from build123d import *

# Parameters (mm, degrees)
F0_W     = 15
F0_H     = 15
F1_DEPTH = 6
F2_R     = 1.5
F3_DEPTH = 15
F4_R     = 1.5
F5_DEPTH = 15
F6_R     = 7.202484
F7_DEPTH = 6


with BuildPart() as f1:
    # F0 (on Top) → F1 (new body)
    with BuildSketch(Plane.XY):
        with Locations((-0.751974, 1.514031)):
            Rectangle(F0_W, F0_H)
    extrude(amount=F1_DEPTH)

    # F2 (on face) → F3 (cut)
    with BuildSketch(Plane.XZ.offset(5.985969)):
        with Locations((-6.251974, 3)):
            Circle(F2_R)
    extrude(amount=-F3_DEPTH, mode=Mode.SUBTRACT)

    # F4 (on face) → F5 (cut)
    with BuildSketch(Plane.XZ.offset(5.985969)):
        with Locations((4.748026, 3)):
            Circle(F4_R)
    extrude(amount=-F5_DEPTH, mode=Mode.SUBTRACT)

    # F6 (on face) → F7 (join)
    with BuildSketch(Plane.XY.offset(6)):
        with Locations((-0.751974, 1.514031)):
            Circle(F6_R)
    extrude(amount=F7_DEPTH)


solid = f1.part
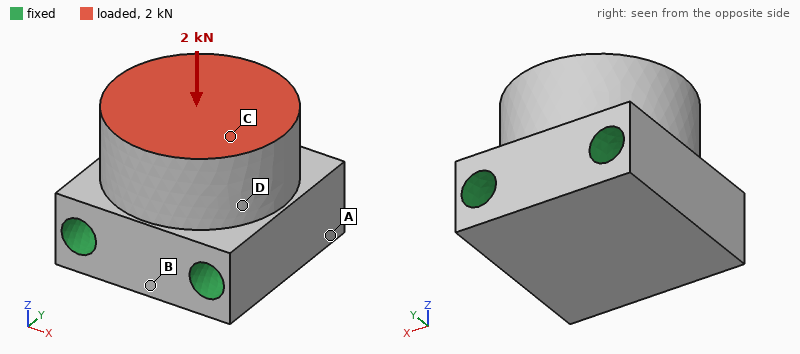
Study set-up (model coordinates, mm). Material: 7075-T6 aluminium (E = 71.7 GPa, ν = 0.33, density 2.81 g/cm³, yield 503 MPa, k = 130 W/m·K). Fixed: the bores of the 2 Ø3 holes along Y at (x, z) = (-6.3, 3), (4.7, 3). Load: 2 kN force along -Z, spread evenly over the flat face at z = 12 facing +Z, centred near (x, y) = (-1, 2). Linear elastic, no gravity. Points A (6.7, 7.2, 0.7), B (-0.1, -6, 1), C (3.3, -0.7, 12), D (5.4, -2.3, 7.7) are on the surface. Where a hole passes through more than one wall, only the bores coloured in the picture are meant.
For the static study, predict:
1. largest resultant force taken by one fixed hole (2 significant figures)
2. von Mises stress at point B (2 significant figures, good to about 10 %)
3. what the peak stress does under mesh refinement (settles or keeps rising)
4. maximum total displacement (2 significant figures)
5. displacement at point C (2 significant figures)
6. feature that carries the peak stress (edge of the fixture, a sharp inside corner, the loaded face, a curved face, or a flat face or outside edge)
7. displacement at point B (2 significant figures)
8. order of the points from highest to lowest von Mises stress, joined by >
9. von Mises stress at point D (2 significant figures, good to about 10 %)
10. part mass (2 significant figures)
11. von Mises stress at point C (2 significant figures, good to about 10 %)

1.0 kN
3.9 MPa
keeps rising
1.8 µm
1.5 µm
edge of the fixture
0.66 µm
D > C > B > A
16 MPa
5.9 g
13 MPa
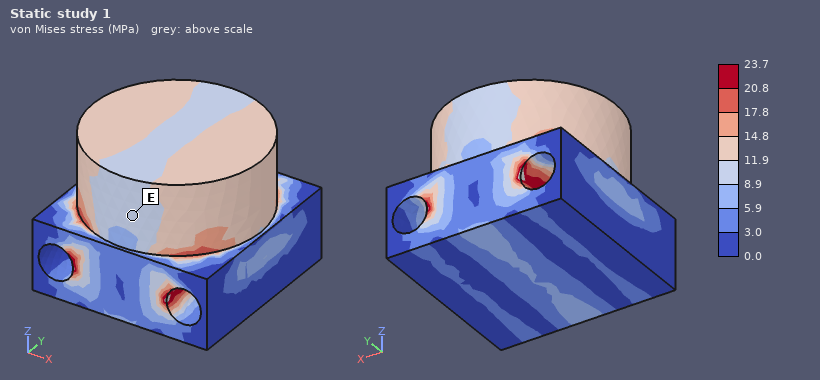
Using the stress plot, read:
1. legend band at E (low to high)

8.9 to 11.9 MPa
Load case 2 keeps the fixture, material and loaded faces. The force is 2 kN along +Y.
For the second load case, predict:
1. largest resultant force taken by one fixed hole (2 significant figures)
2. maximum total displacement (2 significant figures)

1.0 kN
9.2 µm
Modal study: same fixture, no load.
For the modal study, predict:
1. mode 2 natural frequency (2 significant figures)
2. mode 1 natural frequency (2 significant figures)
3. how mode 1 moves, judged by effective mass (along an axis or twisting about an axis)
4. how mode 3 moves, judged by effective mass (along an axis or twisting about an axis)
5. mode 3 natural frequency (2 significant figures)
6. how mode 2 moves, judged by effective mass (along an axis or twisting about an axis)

84 kHz
70 kHz
along Y
twisting about Z
100 kHz
along X
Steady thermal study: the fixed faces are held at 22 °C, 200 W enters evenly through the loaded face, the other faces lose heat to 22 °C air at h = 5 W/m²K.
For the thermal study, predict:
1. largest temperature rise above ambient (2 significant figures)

80 K
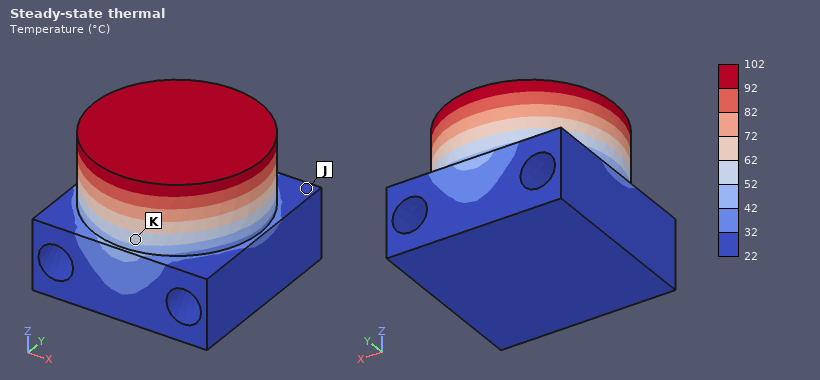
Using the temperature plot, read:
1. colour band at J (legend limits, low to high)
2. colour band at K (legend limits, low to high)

22 to 32 °C
52 to 62 °C
